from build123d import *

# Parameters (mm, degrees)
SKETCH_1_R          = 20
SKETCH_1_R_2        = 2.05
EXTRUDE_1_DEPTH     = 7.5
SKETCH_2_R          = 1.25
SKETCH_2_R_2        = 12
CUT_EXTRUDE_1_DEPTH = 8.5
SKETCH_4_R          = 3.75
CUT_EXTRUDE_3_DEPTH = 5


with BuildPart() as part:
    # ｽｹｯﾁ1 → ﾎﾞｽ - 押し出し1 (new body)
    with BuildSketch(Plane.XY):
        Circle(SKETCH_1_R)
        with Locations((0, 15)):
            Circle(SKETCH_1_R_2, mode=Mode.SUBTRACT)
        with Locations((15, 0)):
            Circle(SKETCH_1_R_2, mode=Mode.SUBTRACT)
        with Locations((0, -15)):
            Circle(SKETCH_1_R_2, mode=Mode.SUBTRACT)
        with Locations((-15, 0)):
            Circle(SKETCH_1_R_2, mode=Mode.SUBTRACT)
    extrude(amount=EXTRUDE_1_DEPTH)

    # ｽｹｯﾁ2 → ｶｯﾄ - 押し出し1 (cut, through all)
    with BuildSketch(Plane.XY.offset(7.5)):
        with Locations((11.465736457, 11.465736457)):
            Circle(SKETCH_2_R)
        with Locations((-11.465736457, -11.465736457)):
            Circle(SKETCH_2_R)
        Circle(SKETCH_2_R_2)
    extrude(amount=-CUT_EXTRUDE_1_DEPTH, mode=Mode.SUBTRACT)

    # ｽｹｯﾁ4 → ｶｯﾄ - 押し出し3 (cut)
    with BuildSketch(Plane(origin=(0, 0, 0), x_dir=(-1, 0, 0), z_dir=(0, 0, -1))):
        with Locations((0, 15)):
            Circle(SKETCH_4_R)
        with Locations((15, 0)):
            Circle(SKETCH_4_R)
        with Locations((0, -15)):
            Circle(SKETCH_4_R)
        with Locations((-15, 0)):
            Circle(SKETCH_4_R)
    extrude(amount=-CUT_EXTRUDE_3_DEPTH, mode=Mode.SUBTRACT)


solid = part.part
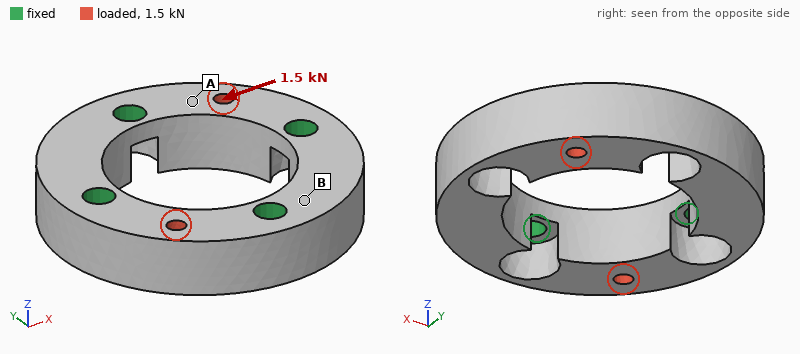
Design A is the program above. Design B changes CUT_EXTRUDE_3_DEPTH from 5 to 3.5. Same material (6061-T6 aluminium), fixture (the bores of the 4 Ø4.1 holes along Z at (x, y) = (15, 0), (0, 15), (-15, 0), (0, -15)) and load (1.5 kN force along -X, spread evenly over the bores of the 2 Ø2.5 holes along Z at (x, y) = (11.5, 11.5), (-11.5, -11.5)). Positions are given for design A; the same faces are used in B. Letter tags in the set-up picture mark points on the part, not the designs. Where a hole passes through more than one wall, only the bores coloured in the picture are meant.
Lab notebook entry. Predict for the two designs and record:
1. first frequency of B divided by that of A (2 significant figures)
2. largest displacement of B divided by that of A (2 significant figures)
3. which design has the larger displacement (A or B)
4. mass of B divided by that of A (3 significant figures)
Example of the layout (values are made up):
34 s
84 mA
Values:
1.5
0.49
A
1.03
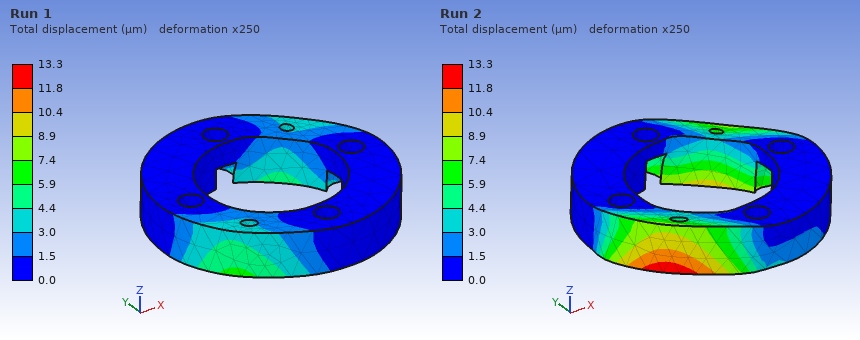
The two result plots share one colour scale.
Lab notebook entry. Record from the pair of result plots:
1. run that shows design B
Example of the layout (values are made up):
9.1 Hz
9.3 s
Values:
Run 1
